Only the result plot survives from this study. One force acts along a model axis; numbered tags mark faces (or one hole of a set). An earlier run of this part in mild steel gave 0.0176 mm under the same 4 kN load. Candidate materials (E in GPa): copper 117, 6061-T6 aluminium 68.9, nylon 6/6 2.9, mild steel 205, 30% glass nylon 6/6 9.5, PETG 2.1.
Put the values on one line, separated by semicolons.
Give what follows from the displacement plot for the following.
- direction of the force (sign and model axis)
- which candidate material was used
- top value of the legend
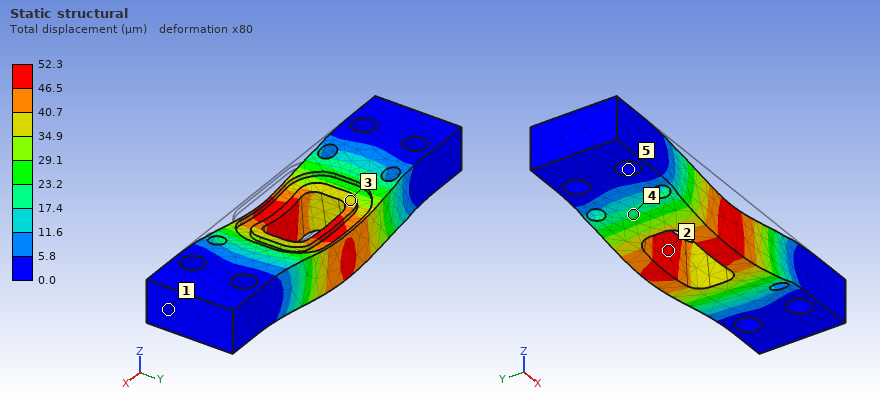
-Z; 6061-T6 aluminium; 52.3 µm
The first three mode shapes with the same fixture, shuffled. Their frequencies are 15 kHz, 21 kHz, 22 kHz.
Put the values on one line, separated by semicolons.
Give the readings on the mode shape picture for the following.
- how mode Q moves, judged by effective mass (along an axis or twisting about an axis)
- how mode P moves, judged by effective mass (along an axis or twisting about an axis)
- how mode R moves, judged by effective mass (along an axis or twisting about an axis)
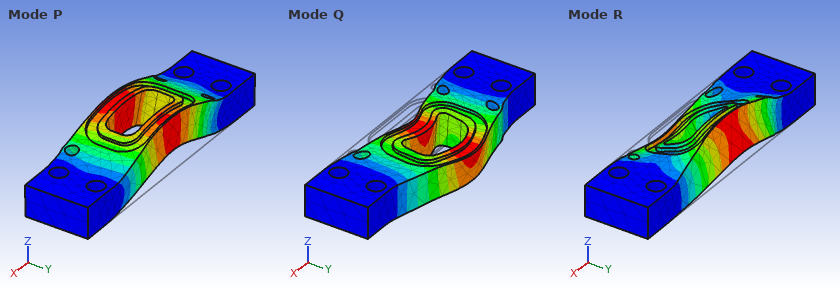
along Y; along Z; twisting about X
